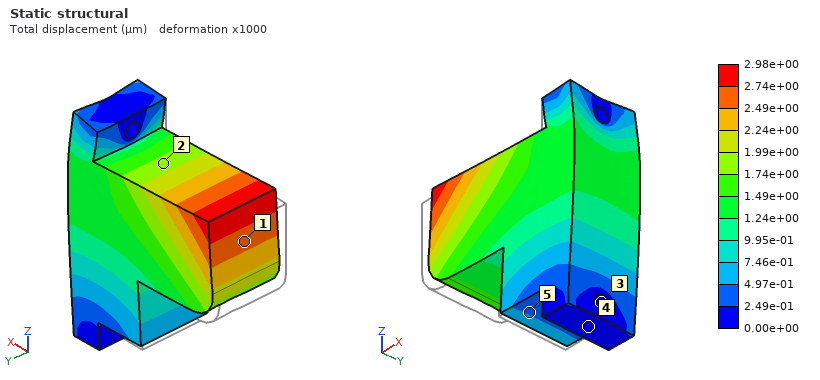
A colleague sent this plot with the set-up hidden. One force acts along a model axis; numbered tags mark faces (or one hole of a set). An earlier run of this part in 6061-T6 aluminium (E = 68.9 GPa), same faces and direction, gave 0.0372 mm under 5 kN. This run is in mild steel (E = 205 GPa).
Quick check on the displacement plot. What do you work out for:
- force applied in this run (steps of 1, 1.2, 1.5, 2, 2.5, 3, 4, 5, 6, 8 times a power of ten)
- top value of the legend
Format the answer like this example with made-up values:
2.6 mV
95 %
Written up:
1.2 kN
2.98e+00 µm
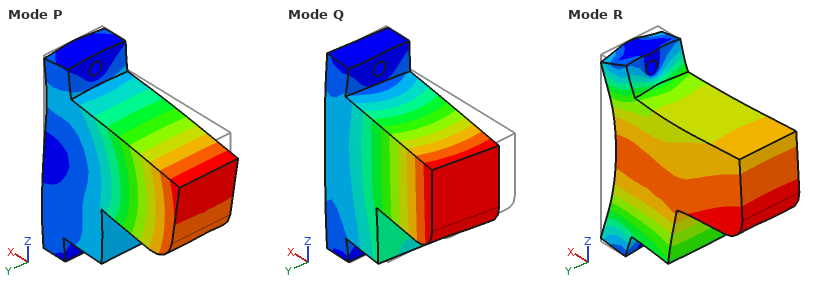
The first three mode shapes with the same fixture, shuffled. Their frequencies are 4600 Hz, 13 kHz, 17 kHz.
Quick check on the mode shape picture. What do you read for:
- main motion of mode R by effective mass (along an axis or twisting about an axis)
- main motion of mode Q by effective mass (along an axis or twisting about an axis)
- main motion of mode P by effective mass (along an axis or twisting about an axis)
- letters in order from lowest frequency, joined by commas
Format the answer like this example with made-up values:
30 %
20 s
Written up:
along X
along Y
along Z
Q, P, R
